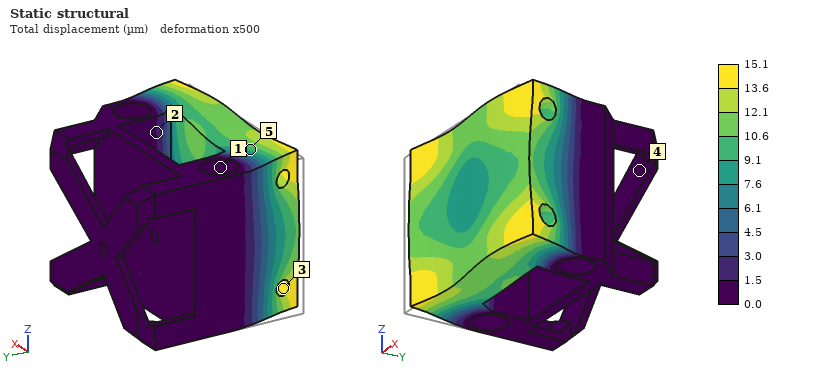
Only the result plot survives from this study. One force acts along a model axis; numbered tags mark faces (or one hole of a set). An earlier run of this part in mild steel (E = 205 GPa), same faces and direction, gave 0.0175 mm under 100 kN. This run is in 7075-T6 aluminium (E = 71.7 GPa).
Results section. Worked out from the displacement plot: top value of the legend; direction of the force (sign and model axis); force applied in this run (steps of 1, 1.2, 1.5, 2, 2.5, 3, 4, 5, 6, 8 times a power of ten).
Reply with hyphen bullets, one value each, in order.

- 15.1 µm
- +X
- 30 kN
